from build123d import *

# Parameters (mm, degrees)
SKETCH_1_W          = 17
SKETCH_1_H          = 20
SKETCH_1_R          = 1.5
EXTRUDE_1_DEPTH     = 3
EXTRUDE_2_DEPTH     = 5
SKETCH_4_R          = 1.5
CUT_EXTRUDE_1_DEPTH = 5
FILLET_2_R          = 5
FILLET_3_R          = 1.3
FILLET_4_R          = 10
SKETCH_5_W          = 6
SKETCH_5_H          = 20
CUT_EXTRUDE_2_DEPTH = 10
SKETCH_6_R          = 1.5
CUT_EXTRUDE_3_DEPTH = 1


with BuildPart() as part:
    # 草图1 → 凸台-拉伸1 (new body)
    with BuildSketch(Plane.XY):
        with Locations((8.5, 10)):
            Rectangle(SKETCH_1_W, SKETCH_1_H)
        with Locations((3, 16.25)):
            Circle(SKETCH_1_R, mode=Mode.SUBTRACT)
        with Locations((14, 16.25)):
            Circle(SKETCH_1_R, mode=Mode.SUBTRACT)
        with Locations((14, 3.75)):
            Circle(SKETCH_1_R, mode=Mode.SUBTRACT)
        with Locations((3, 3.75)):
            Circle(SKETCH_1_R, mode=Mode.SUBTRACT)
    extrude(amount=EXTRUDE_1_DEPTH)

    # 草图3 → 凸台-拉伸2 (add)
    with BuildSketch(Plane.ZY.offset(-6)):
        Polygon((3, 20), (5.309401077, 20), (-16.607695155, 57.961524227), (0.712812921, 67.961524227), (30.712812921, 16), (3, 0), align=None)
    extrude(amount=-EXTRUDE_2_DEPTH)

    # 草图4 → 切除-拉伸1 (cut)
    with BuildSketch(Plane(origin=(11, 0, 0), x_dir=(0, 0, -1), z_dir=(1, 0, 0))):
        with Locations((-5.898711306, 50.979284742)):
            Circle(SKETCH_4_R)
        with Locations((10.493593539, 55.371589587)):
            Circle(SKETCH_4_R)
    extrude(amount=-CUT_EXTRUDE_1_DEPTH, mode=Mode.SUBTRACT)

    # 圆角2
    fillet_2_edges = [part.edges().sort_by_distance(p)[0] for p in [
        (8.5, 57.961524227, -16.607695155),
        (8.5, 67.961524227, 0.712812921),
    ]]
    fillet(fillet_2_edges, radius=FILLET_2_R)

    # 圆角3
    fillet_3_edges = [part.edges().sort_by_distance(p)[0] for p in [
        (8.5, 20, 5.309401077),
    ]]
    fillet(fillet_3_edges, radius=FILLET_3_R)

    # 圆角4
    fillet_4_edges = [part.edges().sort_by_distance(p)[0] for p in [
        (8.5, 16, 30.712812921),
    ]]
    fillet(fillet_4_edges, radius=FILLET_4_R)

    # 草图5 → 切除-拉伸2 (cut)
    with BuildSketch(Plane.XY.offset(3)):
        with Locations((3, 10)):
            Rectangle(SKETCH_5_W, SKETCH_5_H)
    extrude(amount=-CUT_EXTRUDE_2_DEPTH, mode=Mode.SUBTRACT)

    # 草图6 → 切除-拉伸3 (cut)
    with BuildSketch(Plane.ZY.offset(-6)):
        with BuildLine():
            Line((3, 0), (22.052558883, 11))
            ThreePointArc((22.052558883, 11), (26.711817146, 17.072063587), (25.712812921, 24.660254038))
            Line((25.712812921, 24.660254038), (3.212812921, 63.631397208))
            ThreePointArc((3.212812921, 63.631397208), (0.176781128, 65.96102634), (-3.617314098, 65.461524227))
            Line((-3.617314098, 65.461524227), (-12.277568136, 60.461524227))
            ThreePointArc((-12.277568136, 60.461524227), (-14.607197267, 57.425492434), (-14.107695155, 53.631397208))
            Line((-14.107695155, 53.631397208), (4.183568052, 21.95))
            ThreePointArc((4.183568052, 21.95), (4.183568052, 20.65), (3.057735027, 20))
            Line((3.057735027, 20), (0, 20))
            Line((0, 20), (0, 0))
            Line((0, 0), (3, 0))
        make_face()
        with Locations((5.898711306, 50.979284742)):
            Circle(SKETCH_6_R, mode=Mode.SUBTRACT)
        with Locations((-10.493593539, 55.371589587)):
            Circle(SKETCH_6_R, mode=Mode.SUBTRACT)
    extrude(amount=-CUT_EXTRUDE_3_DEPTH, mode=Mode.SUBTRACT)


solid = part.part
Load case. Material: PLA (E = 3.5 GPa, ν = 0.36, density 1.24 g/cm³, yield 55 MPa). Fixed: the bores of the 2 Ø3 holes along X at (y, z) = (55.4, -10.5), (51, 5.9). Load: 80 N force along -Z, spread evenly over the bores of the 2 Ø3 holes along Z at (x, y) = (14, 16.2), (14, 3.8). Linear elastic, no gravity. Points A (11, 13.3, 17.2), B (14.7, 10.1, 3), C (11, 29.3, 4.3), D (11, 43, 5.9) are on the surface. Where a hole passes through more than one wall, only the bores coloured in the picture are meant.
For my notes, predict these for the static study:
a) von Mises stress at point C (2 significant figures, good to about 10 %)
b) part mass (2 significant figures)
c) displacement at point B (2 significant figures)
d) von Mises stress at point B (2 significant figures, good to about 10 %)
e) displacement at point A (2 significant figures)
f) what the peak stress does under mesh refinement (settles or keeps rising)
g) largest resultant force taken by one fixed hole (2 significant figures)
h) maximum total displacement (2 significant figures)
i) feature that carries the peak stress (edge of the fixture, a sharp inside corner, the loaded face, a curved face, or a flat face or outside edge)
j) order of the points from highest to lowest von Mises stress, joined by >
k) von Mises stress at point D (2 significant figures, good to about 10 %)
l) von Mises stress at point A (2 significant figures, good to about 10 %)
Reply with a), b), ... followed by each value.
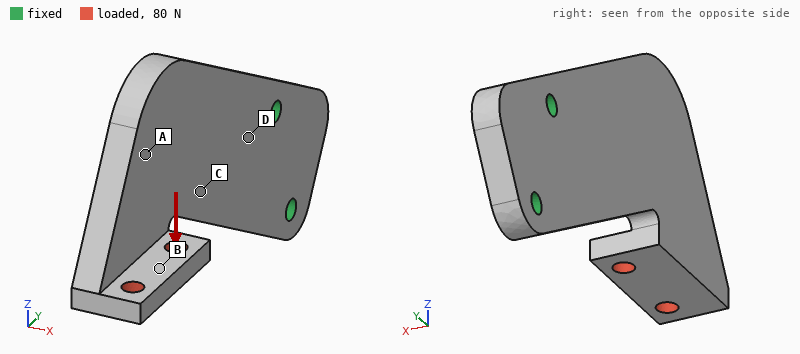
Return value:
a) 12 MPa
b) 7.0 g
c) 0.54 mm
d) 2.7 MPa
e) 0.43 mm
f) keeps rising
g) 200 N
h) 0.79 mm
i) edge of the fixture
j) C > D > A > B
k) 8.5 MPa
l) 5.3 MPa
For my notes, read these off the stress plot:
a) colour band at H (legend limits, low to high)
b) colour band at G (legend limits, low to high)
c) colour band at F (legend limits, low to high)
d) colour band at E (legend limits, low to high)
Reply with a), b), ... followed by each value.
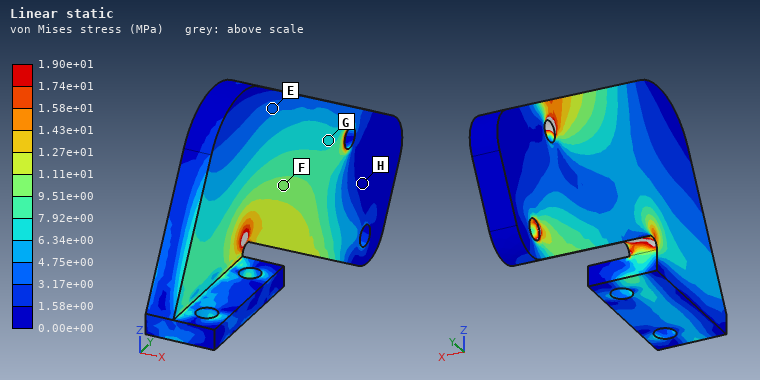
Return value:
a) 0.00e+00 to 1.58e+00 MPa
b) 6.34e+00 to 7.92e+00 MPa
c) 9.51e+00 to 1.11e+01 MPa
d) 3.17e+00 to 4.75e+00 MPa
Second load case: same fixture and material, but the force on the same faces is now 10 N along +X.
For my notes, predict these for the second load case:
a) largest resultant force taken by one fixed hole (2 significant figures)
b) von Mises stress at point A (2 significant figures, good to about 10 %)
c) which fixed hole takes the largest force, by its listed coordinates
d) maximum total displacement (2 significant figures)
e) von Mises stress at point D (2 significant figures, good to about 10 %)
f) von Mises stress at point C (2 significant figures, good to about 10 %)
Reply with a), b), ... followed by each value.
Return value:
a) 14 N
b) 1.5 MPa
c) (51, 5.9)
d) 0.95 mm
e) 5.8 MPa
f) 4.5 MPa
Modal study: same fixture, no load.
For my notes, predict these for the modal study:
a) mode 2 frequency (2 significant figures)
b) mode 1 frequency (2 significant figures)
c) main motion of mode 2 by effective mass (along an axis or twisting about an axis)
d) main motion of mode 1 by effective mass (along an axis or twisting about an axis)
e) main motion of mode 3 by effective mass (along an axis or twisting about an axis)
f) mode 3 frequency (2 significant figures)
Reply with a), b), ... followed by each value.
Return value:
a) 1200 Hz
b) 400 Hz
c) twisting about Y
d) along X
e) along Z
f) 1600 Hz
